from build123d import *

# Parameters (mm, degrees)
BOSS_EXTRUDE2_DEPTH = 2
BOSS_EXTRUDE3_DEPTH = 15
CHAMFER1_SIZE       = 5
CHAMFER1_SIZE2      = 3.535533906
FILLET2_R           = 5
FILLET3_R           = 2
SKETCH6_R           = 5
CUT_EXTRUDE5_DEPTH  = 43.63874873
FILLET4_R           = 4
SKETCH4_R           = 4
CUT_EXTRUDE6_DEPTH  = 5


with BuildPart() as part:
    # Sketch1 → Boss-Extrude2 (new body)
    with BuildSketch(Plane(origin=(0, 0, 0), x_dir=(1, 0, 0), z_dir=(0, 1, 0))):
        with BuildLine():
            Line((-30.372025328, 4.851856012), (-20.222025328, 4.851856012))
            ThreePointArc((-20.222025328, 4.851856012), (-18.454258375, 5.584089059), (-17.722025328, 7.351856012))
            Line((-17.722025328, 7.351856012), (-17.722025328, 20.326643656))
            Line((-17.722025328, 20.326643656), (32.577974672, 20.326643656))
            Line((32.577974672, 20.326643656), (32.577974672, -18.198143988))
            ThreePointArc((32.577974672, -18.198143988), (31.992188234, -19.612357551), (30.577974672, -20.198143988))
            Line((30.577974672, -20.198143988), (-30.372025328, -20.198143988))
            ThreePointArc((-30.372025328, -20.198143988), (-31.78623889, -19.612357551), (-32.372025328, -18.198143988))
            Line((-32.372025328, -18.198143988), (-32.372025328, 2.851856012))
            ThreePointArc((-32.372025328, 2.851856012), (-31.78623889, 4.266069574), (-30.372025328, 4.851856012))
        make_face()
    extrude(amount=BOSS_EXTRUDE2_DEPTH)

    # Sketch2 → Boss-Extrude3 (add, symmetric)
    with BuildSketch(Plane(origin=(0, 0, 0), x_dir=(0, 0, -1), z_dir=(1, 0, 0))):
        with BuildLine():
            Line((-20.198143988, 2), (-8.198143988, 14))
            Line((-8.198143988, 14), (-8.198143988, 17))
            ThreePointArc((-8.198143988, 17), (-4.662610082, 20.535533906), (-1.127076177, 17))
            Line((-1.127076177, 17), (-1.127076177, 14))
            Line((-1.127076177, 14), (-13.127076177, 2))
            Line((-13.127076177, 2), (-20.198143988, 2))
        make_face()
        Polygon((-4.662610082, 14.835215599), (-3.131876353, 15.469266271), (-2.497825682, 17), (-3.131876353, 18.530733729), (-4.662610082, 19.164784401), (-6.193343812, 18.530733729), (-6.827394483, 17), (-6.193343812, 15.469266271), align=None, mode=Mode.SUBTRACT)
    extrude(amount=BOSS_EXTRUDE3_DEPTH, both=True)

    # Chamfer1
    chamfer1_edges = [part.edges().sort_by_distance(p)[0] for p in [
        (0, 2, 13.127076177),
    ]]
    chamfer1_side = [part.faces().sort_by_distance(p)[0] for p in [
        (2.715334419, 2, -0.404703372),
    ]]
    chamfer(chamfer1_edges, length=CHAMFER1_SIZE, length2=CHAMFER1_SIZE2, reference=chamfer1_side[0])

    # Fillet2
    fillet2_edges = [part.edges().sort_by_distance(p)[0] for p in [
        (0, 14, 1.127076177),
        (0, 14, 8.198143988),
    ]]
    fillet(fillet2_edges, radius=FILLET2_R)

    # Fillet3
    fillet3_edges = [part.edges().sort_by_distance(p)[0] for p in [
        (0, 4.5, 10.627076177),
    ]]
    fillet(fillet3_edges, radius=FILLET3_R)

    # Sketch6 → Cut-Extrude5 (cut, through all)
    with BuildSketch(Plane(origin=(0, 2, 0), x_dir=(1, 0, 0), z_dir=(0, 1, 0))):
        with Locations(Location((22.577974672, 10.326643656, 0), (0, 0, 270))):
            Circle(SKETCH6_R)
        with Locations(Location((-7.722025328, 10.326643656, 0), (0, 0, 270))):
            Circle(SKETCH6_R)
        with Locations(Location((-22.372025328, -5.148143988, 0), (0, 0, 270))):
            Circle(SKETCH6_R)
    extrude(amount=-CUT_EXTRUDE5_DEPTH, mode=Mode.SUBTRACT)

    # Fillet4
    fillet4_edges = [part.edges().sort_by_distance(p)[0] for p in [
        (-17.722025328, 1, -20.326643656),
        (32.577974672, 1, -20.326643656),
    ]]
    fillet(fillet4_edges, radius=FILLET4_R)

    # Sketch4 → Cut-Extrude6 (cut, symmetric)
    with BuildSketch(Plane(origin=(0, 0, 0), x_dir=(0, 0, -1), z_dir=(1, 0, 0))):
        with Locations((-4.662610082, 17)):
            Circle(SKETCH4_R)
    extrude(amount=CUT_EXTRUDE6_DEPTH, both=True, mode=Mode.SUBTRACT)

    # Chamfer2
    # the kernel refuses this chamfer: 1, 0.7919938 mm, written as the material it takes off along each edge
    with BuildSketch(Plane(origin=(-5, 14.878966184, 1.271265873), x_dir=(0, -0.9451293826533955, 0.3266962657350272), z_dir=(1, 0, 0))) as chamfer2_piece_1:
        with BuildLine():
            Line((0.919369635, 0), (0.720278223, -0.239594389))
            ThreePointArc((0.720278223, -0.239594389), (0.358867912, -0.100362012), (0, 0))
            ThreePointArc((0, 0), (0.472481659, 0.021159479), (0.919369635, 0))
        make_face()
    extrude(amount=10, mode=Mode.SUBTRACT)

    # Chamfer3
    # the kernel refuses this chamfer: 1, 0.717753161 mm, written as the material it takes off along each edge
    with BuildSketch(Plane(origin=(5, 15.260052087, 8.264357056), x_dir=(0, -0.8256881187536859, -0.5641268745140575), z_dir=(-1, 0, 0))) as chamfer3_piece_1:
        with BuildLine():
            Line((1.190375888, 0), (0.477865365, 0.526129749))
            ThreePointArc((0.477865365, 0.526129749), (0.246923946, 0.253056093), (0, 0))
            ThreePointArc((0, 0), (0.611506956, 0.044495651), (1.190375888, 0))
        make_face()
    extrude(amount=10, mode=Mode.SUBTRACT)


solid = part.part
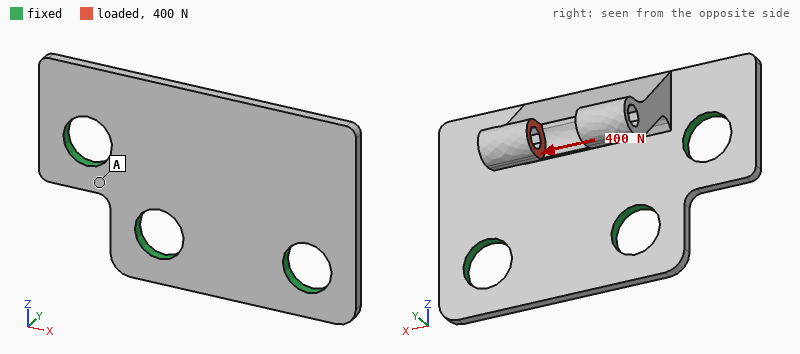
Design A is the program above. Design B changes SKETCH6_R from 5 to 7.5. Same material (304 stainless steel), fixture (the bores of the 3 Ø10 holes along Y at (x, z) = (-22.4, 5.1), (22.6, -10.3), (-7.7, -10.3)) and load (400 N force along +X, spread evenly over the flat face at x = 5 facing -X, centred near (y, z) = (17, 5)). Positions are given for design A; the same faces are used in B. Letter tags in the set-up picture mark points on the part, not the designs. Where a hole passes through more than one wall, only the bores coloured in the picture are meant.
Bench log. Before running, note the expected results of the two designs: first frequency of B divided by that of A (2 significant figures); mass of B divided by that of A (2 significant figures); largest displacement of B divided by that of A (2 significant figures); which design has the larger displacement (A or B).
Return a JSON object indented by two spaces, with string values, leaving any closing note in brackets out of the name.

{
  "first frequency of B divided by that of A": "1.3",
  "mass of B divided by that of A": "0.92",
  "largest displacement of B divided by that of A": "0.68",
  "which design has the larger displacement": "A"
}
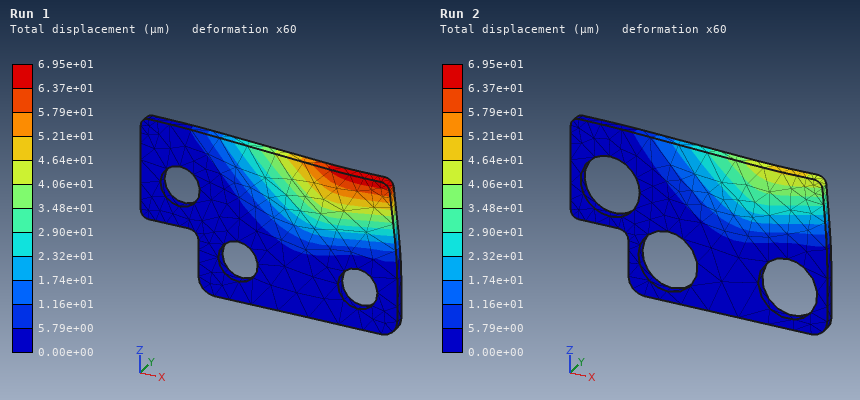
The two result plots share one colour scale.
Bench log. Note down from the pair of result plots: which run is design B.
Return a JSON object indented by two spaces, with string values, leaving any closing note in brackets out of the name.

{
  "which run is design B": "Run 2"
}
